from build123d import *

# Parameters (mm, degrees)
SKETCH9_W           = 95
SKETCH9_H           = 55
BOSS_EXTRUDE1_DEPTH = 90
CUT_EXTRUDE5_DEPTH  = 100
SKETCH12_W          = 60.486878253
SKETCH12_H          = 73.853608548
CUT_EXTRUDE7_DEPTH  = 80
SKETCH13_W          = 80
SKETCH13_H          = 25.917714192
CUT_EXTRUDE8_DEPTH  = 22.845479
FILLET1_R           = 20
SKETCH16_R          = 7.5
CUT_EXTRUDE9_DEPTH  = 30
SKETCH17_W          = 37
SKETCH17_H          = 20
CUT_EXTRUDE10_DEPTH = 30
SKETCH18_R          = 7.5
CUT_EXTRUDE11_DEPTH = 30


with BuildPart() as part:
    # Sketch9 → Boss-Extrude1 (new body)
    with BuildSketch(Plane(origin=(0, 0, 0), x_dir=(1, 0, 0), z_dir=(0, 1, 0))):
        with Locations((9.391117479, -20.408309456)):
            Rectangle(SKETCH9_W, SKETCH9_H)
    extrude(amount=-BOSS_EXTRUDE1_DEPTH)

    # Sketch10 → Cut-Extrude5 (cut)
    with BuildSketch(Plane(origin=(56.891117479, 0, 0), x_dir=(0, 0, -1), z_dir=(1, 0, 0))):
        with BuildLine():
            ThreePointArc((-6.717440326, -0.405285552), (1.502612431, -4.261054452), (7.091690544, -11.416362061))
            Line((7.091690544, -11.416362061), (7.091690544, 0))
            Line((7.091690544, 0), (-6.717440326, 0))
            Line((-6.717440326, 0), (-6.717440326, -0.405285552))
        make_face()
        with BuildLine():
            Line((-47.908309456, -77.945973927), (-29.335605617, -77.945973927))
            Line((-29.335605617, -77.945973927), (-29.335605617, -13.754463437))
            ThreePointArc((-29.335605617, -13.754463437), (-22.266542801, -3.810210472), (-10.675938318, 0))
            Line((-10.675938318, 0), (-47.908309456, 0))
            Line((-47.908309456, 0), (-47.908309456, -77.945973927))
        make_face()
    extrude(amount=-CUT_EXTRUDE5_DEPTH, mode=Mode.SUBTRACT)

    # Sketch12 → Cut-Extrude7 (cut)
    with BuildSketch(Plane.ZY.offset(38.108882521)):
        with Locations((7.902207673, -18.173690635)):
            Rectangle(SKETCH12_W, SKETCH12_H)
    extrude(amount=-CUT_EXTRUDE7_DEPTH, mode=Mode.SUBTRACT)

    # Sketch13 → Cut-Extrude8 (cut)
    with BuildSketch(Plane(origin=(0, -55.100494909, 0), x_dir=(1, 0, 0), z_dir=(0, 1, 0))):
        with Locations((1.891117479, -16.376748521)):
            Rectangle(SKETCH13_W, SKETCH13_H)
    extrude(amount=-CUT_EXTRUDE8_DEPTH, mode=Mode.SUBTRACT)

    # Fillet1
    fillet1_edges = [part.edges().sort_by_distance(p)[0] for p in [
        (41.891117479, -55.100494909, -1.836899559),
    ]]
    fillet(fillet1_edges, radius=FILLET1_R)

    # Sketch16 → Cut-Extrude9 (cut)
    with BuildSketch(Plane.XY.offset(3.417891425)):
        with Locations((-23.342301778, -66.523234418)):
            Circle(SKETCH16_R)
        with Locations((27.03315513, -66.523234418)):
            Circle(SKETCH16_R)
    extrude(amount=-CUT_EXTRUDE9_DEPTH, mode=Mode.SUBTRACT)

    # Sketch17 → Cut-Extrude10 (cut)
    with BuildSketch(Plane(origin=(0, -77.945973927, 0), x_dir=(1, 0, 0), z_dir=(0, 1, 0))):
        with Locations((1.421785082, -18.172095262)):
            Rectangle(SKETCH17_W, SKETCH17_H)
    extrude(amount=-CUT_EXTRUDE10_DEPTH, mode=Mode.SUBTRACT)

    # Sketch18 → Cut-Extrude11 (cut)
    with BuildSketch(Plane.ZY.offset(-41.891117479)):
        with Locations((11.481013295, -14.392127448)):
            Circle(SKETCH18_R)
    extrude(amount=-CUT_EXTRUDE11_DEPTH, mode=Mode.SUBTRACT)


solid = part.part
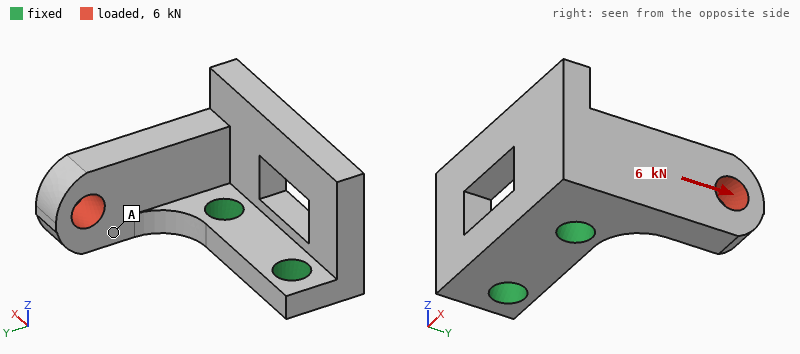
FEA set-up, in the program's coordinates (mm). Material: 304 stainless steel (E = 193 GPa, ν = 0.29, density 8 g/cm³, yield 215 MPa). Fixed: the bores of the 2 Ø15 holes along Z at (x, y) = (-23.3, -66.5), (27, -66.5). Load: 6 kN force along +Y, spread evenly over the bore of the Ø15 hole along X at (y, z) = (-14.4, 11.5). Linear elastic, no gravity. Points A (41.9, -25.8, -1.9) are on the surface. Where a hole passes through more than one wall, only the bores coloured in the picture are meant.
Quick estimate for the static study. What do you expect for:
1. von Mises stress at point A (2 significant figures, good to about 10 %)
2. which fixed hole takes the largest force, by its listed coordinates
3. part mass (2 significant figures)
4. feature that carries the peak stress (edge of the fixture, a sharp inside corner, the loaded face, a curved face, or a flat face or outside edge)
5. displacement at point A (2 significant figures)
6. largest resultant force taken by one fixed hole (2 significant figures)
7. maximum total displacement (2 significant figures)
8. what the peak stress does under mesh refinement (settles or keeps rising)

14 MPa
(27, -66.5)
870 g
edge of the fixture
25 µm
6.9 kN
46 µm
keeps rising
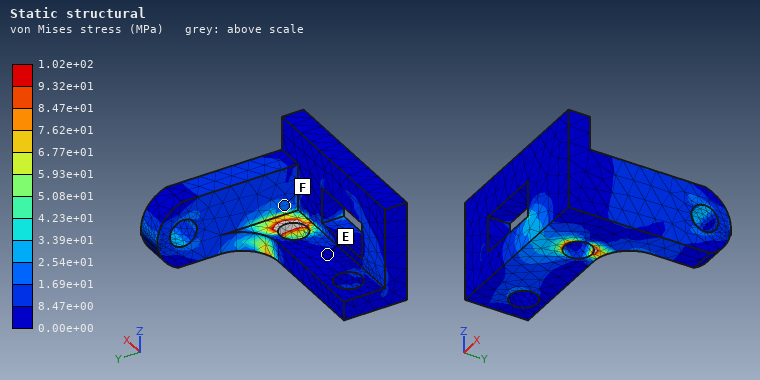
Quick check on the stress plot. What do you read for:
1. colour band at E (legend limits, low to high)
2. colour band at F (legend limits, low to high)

0.00e+00 to 8.47e+00 MPa
1.69e+01 to 2.54e+01 MPa
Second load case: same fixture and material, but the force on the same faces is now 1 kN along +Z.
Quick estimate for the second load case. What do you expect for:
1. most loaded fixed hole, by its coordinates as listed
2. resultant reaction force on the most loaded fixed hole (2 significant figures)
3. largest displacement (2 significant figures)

(27, -66.5)
1.0 kN
35 µm
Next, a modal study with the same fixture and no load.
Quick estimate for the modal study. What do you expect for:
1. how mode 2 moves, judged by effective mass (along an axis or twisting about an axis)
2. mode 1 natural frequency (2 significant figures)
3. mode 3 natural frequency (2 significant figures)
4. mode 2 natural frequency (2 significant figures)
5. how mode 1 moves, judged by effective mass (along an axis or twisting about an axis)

along X
2100 Hz
3400 Hz
2800 Hz
along Y
